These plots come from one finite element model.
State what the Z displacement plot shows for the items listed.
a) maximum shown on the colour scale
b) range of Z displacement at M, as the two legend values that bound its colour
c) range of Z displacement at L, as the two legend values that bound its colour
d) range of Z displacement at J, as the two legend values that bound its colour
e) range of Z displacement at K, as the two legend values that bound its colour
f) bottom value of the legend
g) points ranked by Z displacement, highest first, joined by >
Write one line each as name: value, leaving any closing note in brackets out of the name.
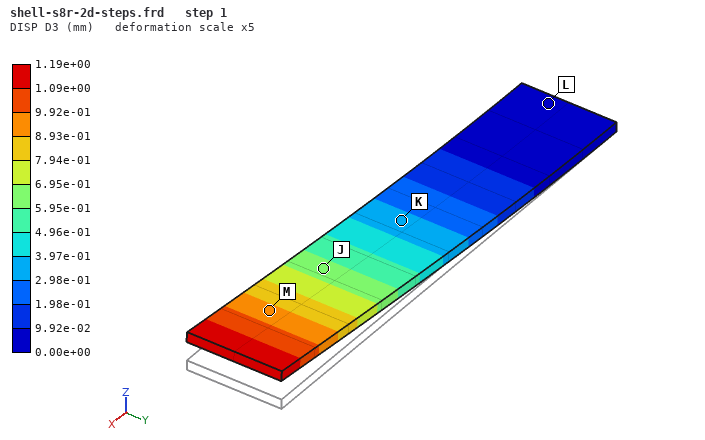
maximum shown on the colour scale: 1.19e+00 mm
range of Z displacement at M, as the two legend values that bound its colour: 8.93e-01 to 9.92e-01 mm
range of Z displacement at L, as the two legend values that bound its colour: 0.00e+00 to 9.92e-02 mm
range of Z displacement at J, as the two legend values that bound its colour: 5.95e-01 to 6.95e-01 mm
range of Z displacement at K, as the two legend values that bound its colour: 2.98e-01 to 3.97e-01 mm
bottom value of the legend: 0.00e+00 mm
points ranked by Z displacement, highest first, joined by >: M > J > K > L
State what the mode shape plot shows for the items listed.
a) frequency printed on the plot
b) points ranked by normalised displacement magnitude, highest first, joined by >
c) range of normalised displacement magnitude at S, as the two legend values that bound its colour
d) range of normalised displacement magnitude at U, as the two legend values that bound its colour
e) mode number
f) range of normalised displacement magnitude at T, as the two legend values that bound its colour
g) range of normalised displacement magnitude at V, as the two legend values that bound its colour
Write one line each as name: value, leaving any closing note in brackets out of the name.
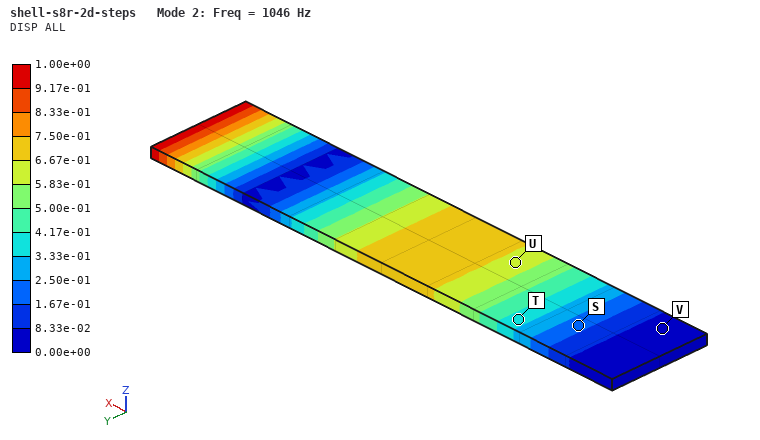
frequency printed on the plot: 1046 Hz
points ranked by normalised displacement magnitude, highest first, joined by >: U > T > S > V
range of normalised displacement magnitude at S, as the two legend values that bound its colour: 1.67e-01 to 2.50e-01
range of normalised displacement magnitude at U, as the two legend values that bound its colour: 5.83e-01 to 6.67e-01
mode number: 2
range of normalised displacement magnitude at T, as the two legend values that bound its colour: 3.33e-01 to 4.17e-01
range of normalised displacement magnitude at V, as the two legend values that bound its colour: 0.00e+00 to 8.33e-02
